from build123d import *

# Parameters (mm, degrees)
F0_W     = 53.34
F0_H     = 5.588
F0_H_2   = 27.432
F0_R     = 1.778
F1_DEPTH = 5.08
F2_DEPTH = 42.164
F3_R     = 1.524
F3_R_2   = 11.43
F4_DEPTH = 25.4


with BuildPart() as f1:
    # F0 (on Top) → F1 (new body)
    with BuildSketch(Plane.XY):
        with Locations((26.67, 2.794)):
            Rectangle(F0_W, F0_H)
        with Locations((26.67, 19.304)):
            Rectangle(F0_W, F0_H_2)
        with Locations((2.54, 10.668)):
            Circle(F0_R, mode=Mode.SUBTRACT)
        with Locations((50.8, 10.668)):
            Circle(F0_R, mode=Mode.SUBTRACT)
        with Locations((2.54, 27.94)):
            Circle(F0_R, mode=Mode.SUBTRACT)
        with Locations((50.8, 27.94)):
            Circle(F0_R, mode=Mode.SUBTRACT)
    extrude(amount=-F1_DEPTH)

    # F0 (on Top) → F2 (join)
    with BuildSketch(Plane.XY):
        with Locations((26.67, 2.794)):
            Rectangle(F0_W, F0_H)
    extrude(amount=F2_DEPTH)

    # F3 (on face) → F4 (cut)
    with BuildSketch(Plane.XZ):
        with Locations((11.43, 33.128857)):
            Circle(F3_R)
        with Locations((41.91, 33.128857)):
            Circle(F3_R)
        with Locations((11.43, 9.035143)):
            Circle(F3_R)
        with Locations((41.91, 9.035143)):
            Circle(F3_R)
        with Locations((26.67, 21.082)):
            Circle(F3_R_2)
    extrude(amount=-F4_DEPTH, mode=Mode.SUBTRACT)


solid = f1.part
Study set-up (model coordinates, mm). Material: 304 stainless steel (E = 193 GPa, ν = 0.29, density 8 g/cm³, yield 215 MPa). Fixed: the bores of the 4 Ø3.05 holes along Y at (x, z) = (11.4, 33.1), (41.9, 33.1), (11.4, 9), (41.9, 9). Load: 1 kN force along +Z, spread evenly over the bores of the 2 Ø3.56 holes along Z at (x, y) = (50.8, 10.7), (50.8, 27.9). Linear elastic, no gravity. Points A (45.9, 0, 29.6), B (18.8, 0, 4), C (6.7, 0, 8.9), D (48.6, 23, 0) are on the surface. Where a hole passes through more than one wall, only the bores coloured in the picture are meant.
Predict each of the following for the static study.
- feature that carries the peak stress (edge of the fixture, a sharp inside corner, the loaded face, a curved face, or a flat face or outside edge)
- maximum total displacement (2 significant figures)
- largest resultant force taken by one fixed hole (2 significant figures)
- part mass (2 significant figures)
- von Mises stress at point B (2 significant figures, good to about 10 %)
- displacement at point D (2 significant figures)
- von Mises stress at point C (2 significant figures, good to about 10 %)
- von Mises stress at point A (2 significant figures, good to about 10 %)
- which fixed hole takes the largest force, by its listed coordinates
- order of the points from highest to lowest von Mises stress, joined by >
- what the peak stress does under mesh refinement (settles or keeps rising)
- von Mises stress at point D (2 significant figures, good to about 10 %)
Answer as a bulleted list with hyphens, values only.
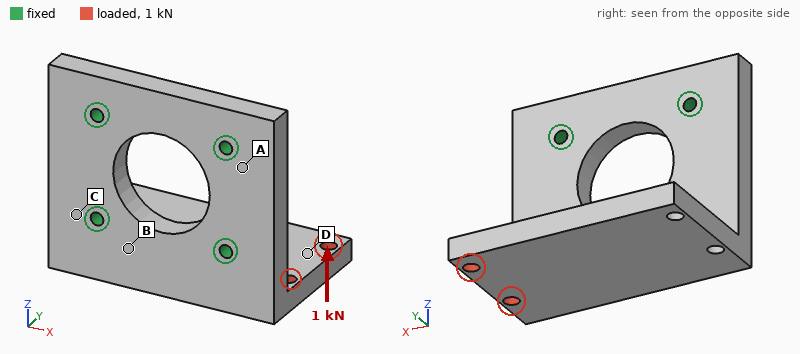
- edge of the fixture
- 0.13 mm
- 940 N
- 150 g
- 42 MPa
- 0.076 mm
- 26 MPa
- 10 MPa
- (41.9, 9)
- D > B > C > A
- keeps rising
- 55 MPa
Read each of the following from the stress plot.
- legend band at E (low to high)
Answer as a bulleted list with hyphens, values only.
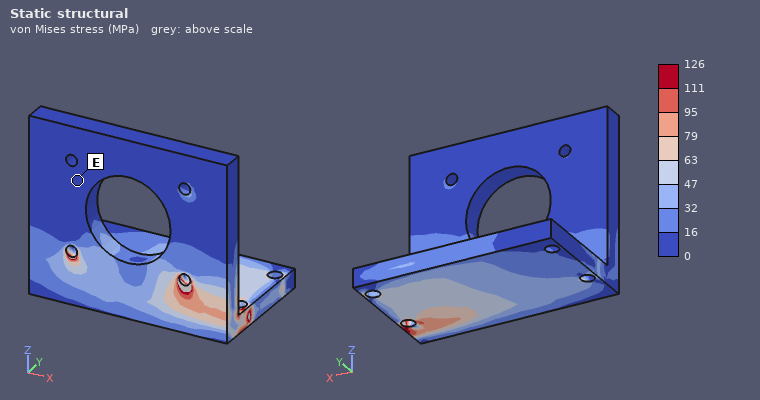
- 0 to 16 MPa
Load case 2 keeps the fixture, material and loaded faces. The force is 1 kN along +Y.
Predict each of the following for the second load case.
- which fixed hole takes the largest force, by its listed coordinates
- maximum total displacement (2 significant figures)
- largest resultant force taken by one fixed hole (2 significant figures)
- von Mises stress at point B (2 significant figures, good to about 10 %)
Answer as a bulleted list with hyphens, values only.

- (41.9, 9)
- 37 µm
- 1.3 kN
- 23 MPa
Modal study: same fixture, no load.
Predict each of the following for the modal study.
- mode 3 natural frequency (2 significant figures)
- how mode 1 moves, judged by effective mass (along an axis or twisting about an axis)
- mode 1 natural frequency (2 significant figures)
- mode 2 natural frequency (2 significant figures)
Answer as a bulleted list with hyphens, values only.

- 8100 Hz
- along Z
- 2900 Hz
- 5500 Hz
